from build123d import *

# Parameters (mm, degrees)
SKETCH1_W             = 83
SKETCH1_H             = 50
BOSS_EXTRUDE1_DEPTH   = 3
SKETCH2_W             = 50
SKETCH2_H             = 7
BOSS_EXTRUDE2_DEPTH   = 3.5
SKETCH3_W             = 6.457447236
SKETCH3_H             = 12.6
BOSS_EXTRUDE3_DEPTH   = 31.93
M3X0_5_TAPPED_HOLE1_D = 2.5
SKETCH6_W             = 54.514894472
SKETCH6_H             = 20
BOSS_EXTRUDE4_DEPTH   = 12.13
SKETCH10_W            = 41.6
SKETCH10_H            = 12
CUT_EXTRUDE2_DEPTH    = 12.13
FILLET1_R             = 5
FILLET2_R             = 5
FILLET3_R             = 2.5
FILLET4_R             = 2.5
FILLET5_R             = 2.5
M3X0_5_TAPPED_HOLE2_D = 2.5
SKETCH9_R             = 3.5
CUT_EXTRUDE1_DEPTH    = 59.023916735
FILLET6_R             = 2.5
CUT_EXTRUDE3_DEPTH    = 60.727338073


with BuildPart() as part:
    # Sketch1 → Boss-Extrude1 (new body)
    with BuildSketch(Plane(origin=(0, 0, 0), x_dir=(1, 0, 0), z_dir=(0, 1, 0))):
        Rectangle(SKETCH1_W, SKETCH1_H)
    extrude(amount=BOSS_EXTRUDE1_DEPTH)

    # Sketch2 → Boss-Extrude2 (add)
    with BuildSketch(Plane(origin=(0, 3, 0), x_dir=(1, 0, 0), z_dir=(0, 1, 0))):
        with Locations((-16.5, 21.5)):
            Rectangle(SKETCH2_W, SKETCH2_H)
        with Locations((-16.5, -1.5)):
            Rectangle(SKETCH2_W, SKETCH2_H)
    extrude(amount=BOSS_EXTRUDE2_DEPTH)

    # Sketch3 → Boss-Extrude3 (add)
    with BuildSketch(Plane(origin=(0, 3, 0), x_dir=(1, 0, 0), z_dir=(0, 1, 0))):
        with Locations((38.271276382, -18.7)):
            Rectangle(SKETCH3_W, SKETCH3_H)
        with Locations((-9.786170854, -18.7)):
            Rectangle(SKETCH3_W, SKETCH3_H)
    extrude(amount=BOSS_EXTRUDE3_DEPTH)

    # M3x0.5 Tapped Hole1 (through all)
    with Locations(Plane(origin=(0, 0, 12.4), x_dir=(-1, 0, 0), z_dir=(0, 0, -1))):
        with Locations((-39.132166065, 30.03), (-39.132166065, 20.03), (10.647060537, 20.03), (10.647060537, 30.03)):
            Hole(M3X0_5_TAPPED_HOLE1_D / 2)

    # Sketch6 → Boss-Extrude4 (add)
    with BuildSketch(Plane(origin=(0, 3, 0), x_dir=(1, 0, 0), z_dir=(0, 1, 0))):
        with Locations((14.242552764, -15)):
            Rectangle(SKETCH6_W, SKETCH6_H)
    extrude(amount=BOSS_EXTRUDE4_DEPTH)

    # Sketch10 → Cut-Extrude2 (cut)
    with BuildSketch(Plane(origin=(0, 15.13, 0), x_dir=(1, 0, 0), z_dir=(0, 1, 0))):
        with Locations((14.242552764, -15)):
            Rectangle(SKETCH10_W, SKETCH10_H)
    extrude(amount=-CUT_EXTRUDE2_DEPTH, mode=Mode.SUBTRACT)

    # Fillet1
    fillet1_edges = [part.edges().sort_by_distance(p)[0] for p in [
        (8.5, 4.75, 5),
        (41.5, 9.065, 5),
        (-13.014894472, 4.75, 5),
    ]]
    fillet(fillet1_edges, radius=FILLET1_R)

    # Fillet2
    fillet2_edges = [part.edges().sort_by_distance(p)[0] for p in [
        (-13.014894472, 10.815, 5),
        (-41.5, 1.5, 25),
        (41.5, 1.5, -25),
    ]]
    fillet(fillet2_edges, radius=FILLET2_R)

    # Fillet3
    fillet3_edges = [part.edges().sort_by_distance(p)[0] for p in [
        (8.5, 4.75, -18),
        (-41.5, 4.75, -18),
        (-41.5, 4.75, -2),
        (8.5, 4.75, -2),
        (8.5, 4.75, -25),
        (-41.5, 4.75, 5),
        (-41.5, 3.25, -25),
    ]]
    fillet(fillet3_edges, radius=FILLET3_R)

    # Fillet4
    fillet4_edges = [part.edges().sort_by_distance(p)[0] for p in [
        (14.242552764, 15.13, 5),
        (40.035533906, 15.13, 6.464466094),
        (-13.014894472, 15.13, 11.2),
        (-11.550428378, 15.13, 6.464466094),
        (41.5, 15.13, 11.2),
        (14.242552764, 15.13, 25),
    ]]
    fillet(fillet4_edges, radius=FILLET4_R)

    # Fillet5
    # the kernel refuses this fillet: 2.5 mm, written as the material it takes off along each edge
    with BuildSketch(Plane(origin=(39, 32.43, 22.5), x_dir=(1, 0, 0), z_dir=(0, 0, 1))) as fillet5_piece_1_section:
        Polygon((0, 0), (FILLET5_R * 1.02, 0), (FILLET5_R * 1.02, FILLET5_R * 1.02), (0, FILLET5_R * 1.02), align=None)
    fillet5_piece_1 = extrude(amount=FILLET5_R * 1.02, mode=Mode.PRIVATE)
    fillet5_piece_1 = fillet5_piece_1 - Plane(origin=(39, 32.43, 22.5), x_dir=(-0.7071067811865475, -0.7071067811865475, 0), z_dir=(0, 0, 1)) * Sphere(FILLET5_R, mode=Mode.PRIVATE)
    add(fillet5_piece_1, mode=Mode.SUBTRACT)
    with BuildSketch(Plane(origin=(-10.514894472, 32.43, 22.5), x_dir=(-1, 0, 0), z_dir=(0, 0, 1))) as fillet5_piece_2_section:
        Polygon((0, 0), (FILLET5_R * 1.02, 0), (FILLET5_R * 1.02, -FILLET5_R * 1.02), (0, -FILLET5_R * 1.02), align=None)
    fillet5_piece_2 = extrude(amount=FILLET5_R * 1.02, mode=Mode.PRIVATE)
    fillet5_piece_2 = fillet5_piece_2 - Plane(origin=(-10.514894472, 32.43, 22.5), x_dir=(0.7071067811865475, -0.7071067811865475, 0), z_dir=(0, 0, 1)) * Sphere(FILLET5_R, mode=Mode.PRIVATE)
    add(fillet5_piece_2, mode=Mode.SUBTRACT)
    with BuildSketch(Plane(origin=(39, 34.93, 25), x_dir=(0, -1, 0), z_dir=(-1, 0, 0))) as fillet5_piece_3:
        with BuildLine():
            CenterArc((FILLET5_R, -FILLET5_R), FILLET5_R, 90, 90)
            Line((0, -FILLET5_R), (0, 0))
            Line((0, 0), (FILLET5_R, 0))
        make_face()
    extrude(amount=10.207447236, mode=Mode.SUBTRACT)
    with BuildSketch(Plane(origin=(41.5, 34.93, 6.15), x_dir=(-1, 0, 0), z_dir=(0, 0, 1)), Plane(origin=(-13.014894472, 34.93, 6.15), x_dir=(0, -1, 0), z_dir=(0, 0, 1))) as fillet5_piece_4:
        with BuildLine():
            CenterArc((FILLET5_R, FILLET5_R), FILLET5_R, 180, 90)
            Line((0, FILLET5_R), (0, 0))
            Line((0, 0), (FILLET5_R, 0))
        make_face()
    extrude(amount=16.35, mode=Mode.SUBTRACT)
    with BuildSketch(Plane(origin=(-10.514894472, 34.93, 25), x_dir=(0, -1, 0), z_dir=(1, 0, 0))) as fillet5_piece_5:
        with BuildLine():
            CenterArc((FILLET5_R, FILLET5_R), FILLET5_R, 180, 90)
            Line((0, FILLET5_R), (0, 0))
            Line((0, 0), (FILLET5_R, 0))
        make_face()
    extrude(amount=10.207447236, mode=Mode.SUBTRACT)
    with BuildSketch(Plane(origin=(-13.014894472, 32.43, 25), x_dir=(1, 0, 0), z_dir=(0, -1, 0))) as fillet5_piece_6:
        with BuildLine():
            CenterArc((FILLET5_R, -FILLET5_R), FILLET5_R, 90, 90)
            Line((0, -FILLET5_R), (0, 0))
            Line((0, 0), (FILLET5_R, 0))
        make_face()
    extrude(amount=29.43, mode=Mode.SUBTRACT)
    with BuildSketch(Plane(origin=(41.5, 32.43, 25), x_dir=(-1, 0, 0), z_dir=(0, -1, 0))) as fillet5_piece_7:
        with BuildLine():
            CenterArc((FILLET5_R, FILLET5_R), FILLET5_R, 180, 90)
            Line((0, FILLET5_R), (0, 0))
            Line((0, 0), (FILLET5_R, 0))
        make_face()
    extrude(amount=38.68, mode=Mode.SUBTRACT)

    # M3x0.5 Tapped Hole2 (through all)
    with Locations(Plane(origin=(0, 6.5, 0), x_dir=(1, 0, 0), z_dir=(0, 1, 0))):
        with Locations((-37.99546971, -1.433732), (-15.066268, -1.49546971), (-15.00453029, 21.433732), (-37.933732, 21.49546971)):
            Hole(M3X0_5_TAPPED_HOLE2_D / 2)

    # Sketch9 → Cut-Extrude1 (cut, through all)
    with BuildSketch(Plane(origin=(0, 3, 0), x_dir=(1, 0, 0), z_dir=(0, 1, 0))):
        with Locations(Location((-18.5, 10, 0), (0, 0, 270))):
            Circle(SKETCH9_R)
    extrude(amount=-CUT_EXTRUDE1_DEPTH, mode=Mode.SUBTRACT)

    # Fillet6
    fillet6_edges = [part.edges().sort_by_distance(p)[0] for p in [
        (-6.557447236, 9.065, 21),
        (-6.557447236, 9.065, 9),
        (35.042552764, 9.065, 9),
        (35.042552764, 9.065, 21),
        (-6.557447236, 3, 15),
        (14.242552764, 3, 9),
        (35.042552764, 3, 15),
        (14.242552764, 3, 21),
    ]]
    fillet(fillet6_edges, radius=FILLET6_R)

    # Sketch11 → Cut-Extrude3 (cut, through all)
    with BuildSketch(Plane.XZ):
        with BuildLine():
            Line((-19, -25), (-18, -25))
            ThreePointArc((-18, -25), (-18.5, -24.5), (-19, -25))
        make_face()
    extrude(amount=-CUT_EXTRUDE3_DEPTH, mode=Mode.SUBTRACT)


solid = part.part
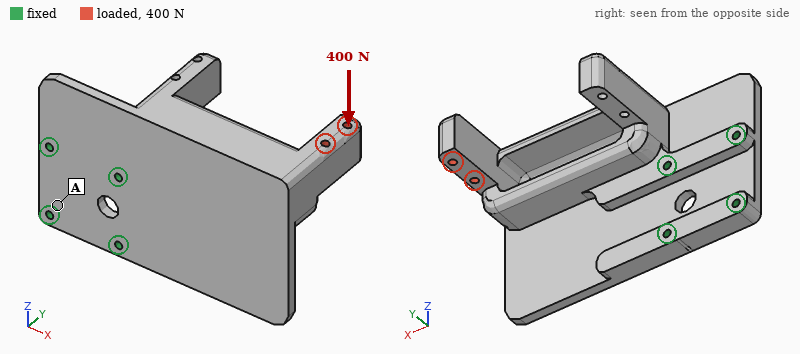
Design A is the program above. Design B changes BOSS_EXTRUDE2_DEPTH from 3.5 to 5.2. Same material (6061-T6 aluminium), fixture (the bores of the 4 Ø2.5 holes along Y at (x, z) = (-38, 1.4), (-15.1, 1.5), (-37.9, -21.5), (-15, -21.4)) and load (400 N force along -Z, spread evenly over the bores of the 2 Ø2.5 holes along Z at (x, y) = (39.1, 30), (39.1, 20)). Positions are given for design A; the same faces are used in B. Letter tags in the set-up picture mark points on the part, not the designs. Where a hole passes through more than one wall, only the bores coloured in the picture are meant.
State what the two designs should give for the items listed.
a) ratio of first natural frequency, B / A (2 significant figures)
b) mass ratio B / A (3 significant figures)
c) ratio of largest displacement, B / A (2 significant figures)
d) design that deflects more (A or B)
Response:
1.3
1.05
0.83
A
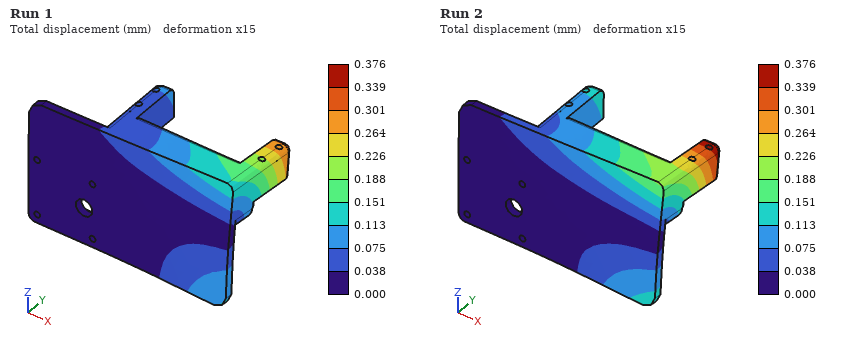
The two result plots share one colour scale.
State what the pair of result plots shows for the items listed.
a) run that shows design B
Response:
Run 1
